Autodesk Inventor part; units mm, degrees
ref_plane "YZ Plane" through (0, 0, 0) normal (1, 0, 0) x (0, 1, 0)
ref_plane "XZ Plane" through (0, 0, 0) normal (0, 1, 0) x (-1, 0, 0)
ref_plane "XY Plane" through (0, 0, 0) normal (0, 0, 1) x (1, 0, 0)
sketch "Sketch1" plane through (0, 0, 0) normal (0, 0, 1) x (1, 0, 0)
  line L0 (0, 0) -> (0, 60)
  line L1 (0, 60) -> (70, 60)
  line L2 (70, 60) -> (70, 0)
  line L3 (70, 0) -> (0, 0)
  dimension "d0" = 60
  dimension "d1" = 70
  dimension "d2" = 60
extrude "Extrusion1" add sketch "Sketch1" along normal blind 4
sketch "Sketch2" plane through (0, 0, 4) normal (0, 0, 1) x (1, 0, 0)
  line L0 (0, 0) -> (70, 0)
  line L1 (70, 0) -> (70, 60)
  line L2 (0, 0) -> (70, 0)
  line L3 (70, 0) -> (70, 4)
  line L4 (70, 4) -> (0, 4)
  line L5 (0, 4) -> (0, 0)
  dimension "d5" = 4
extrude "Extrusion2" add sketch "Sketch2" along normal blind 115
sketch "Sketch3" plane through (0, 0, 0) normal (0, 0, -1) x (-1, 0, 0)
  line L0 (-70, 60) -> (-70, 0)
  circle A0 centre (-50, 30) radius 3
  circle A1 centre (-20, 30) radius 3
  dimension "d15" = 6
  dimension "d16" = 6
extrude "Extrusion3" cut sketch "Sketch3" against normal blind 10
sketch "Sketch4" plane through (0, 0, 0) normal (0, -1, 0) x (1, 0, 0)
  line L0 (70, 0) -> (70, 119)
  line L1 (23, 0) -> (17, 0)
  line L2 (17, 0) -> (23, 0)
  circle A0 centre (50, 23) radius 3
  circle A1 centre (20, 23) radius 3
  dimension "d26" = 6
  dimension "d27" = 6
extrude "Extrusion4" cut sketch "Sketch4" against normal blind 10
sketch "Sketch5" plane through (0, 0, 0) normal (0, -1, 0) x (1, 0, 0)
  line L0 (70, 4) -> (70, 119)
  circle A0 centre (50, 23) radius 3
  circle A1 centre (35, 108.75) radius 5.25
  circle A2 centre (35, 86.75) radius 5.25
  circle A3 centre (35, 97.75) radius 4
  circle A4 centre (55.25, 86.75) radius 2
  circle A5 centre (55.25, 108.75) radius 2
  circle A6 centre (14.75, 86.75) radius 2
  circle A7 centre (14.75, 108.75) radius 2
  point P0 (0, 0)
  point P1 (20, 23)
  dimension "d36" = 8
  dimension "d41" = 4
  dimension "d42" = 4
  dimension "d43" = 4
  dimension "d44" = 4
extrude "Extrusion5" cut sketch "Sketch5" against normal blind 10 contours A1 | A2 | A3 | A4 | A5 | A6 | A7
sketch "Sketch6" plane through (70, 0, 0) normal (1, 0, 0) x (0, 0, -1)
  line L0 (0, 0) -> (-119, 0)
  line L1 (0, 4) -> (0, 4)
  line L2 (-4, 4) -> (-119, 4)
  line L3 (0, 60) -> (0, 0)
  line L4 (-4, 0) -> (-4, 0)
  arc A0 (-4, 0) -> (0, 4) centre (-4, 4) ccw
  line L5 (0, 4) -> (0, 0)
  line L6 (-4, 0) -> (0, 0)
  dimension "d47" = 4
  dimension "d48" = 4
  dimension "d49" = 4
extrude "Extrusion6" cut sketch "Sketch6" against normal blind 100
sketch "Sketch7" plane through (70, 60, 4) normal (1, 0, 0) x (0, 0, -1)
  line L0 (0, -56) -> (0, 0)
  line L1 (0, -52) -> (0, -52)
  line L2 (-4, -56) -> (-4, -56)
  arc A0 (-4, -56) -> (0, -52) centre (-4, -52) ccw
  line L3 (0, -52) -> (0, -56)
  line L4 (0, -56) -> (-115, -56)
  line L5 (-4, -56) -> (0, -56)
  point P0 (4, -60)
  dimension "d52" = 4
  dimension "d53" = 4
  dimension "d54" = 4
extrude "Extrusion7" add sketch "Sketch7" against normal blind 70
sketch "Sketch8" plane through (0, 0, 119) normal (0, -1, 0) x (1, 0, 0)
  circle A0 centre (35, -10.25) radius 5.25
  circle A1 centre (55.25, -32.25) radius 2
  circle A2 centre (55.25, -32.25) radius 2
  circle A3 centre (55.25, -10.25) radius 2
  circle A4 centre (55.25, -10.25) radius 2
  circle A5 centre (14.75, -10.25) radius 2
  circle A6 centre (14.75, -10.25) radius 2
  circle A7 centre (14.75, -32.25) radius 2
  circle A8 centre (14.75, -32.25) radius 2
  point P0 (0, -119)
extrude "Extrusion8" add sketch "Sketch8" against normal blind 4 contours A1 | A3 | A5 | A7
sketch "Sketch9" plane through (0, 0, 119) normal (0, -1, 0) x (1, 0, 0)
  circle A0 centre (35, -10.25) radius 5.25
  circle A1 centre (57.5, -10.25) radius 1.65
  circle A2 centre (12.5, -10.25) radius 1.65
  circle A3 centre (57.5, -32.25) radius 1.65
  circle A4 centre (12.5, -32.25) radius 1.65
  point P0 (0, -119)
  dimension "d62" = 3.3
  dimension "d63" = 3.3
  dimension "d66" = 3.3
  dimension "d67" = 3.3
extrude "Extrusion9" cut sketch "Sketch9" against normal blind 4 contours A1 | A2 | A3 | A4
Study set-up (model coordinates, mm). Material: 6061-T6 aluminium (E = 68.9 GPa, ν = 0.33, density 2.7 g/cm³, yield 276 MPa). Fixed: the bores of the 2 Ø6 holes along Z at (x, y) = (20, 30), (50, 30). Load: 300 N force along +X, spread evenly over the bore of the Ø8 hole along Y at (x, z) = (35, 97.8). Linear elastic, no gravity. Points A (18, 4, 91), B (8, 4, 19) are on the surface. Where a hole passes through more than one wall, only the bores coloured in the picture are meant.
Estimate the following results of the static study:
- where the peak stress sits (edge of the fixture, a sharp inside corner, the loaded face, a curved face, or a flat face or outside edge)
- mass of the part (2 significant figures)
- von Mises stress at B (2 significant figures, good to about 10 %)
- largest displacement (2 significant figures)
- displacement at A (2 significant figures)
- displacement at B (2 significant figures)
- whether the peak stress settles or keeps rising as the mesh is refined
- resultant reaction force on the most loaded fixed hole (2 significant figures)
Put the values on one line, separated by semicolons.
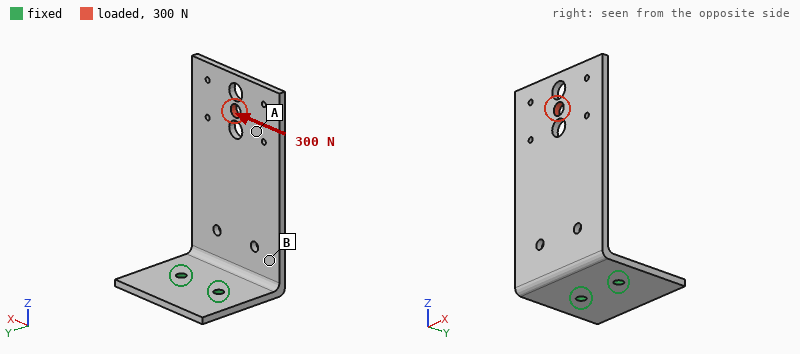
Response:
edge of the fixture; 130 g; 35 MPa; 0.98 mm; 0.72 mm; 0.25 mm; keeps rising; 770 N
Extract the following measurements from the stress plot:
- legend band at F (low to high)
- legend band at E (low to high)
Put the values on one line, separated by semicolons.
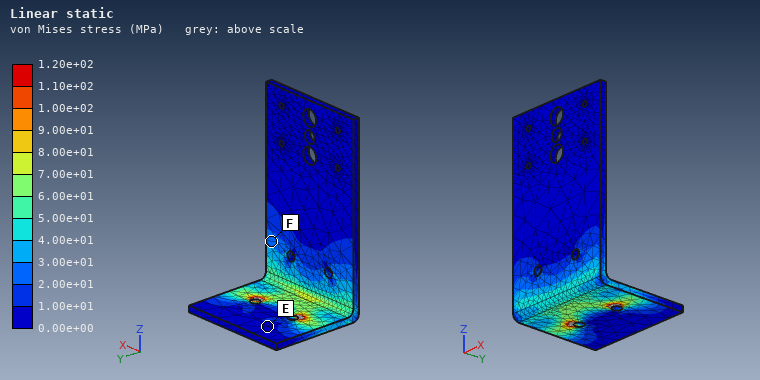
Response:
2.00e+01 to 3.00e+01 MPa; 0.00e+00 to 1.00e+01 MPa
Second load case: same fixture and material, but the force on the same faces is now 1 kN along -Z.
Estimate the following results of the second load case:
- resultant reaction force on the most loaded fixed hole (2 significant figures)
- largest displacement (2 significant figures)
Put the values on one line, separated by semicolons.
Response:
500 N; 1.7 mm
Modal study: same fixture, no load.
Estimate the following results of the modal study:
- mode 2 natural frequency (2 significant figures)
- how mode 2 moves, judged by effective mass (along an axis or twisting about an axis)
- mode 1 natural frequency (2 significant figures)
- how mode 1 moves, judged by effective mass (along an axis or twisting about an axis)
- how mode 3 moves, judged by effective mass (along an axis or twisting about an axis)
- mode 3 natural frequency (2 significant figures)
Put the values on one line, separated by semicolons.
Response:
470 Hz; along X; 190 Hz; along Y; twisting about Z; 860 Hz
